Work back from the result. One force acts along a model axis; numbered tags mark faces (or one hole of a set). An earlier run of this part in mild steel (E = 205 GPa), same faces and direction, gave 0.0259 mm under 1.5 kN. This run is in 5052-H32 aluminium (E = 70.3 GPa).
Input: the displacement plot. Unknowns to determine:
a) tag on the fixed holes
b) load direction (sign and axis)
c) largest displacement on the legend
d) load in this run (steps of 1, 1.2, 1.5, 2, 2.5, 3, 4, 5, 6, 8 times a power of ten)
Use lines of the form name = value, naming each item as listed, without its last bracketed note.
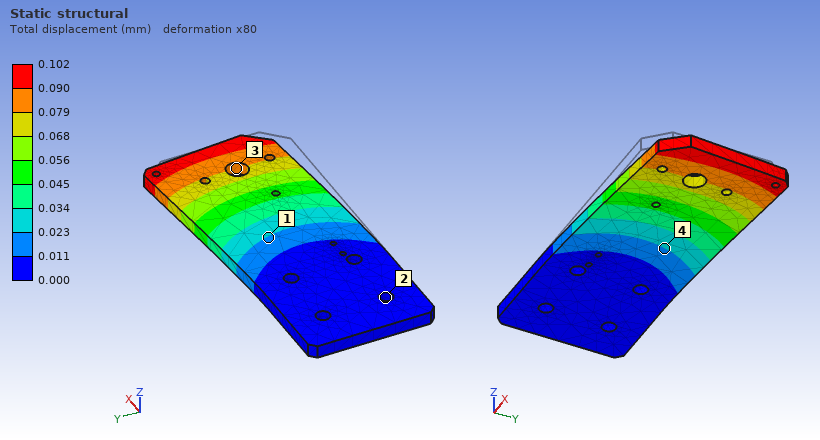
tag on the fixed holes = 2
load direction = +Y
largest displacement on the legend = 0.102 mm
load in this run = 2 kN
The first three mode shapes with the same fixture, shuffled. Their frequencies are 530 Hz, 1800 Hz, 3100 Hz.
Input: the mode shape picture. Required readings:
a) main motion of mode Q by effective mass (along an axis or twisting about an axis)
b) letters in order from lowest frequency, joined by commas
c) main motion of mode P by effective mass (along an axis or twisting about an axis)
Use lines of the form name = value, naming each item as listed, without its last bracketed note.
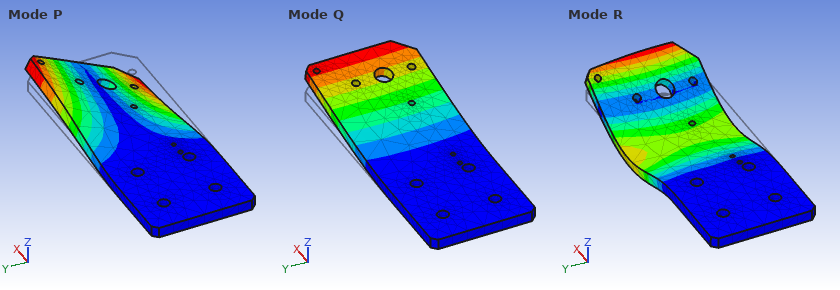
main motion of mode Q by effective mass = along Z
letters in order from lowest frequency, joined by commas = Q, P, R
main motion of mode P by effective mass = twisting about X
